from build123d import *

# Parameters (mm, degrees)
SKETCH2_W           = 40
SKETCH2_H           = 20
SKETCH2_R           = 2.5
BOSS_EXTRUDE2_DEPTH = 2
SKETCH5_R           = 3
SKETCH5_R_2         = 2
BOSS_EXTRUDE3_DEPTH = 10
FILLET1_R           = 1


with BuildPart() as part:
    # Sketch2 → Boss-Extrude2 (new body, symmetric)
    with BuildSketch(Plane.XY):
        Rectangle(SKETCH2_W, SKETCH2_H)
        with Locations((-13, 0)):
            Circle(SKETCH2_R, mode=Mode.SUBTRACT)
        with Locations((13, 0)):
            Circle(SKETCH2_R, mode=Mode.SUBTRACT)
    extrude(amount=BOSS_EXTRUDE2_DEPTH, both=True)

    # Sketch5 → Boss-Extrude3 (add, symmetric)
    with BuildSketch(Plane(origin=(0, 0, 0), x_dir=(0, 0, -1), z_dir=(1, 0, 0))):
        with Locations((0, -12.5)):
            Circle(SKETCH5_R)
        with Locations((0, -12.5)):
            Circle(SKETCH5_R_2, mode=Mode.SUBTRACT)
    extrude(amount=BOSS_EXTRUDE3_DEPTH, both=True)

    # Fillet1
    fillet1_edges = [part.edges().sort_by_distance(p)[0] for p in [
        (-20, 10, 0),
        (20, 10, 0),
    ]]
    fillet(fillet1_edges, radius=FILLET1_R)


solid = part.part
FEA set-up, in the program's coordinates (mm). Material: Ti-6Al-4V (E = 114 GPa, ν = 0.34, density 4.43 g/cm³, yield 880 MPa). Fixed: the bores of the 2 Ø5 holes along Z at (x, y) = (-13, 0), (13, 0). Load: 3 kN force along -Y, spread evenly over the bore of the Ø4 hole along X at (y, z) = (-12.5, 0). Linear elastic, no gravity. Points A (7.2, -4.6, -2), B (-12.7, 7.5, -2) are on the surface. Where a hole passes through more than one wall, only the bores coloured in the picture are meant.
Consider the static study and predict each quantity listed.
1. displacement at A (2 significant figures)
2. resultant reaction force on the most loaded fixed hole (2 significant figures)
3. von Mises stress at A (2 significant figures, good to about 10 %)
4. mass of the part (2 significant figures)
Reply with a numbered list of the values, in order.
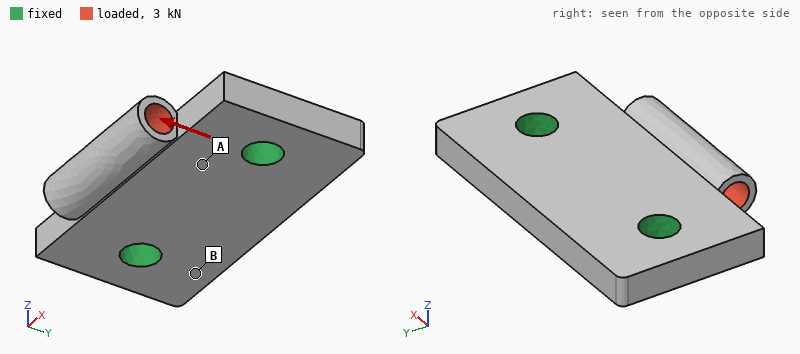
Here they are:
1. 3.0 µm
2. 1.6 kN
3. 39 MPa
4. 15 g
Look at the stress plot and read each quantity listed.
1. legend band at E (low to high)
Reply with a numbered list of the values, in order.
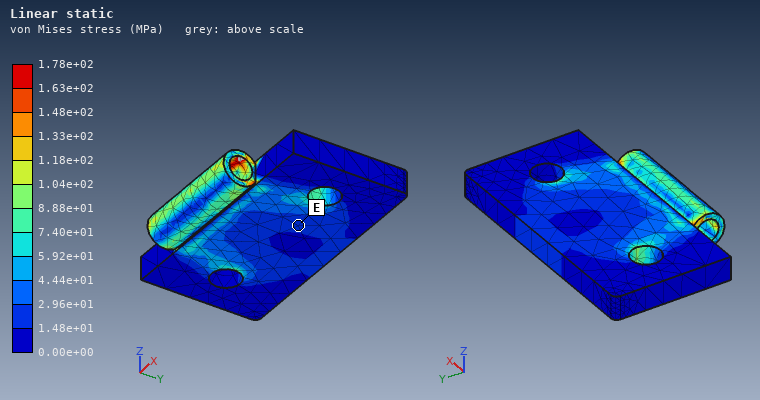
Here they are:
1. 1.48e+01 to 2.96e+01 MPa
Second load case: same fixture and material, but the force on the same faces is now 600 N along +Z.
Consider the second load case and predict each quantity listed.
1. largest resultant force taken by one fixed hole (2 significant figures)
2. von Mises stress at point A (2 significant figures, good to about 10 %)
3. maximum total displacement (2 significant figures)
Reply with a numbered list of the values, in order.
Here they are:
1. 300 N
2. 53 MPa
3. 47 µm
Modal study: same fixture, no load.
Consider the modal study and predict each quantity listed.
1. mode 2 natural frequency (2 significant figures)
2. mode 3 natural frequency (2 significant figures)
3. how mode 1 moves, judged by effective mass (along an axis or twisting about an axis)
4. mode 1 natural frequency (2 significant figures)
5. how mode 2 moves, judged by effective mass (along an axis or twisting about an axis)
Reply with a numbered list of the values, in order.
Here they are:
1. 26 kHz
2. 34 kHz
3. along Z
4. 15 kHz
5. along Z
